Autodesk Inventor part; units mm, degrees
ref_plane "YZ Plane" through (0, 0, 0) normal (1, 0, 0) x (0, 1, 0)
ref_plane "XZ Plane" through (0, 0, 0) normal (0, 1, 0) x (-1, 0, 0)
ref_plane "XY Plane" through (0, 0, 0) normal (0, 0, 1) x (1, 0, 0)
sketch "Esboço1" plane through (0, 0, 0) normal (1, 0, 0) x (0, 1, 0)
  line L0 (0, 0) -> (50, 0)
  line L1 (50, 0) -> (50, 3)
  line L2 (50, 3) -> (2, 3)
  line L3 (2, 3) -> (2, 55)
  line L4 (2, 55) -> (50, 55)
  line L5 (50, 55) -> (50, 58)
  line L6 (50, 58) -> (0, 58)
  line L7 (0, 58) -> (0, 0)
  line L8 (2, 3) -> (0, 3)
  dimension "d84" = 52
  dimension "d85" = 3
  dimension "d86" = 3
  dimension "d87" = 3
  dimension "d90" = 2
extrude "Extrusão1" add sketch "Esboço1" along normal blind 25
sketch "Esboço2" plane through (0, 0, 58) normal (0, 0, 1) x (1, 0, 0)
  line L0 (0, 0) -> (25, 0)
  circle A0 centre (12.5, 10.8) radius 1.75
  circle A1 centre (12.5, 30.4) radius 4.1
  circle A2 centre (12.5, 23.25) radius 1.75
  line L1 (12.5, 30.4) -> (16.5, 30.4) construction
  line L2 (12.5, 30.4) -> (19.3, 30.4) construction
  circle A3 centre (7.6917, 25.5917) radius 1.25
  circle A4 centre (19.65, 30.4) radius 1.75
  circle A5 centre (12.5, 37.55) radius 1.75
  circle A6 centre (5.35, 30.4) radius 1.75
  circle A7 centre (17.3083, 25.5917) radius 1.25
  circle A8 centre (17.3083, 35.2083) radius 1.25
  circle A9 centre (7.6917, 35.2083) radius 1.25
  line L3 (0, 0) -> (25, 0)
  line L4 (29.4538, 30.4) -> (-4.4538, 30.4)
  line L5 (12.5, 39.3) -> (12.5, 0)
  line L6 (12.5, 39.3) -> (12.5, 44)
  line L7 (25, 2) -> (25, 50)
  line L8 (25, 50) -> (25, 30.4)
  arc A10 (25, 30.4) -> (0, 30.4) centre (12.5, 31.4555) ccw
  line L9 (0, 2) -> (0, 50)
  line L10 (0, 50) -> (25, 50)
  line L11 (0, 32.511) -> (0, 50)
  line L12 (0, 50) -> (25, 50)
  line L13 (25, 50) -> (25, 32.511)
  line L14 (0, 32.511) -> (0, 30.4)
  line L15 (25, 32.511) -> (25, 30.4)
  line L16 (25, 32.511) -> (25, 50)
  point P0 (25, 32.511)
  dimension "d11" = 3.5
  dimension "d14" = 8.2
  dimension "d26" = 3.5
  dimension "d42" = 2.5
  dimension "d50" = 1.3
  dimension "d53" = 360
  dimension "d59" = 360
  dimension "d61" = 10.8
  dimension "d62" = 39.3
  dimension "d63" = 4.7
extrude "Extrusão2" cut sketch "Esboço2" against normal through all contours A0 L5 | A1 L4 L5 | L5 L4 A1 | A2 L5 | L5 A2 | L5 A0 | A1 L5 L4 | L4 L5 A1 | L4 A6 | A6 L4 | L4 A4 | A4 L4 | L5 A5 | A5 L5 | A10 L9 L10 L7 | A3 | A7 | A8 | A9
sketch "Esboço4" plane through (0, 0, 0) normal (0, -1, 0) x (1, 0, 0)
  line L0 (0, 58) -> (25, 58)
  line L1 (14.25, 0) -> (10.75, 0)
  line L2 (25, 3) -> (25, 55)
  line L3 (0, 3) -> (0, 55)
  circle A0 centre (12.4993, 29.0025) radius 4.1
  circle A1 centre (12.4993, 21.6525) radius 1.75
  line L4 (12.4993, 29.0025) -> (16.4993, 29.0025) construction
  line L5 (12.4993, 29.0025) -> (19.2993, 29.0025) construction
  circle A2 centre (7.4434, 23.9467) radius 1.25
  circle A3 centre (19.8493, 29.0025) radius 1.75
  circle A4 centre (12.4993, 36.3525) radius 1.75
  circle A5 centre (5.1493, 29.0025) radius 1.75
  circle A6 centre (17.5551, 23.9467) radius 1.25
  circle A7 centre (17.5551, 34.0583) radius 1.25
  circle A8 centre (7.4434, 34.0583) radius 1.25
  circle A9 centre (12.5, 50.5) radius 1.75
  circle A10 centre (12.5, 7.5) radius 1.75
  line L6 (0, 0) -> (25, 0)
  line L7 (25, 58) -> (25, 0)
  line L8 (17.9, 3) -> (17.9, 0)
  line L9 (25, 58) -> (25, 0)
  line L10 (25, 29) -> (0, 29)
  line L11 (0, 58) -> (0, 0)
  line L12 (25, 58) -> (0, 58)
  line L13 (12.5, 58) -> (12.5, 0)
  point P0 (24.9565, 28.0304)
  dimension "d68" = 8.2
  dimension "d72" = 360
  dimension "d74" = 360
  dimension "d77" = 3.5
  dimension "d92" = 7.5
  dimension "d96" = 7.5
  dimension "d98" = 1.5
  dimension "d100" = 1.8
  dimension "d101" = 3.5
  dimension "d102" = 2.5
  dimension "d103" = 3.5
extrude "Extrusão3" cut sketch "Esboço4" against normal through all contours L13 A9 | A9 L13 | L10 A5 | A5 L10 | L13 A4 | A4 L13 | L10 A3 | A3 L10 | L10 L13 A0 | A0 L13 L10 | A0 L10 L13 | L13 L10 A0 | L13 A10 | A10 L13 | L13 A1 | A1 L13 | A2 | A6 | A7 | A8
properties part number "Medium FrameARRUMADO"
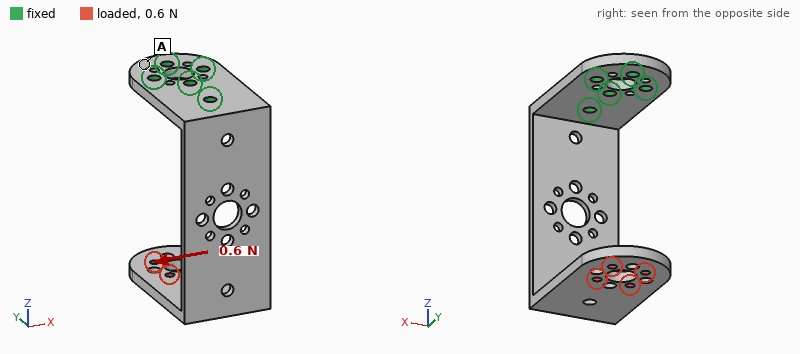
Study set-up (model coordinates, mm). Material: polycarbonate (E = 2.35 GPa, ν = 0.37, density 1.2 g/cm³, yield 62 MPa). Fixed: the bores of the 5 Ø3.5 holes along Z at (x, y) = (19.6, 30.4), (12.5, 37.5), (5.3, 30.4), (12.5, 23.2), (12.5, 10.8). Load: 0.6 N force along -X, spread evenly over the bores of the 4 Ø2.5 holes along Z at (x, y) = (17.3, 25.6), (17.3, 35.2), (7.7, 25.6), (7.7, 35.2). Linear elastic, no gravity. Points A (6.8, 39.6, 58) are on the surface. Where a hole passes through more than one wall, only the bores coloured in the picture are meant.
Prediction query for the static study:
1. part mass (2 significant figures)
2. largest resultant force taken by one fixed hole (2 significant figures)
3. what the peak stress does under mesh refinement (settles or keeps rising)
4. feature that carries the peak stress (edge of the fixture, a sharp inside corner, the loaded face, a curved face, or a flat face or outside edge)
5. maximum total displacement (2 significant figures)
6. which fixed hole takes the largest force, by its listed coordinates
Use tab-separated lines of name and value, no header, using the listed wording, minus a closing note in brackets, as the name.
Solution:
part mass	9.4 g
largest resultant force taken by one fixed hole	0.36 N
what the peak stress does under mesh refinement	keeps rising
feature that carries the peak stress	edge of the fixture
maximum total displacement	0.89 mm
which fixed hole takes the largest force, by its listed coordinates	(12.5, 23.2)
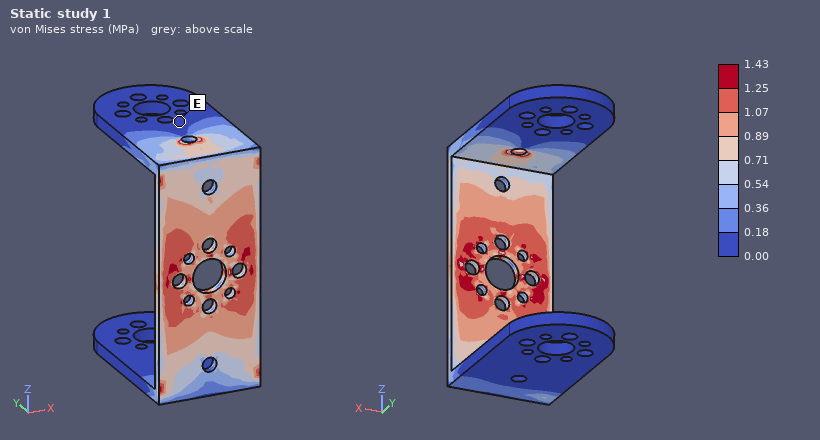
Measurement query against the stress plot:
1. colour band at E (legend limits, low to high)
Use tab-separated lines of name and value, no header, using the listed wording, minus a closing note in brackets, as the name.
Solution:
colour band at E	0.00 to 0.18 MPa
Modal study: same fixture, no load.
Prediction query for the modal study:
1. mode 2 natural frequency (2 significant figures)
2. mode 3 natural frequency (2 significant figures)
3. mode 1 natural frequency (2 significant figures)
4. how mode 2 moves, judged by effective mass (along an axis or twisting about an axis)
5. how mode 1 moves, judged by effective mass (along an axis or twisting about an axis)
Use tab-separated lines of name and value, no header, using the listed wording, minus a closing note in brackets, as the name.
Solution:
mode 2 natural frequency	100 Hz
mode 3 natural frequency	200 Hz
mode 1 natural frequency	52 Hz
how mode 2 moves, judged by effective mass	along X
how mode 1 moves, judged by effective mass	along Y
